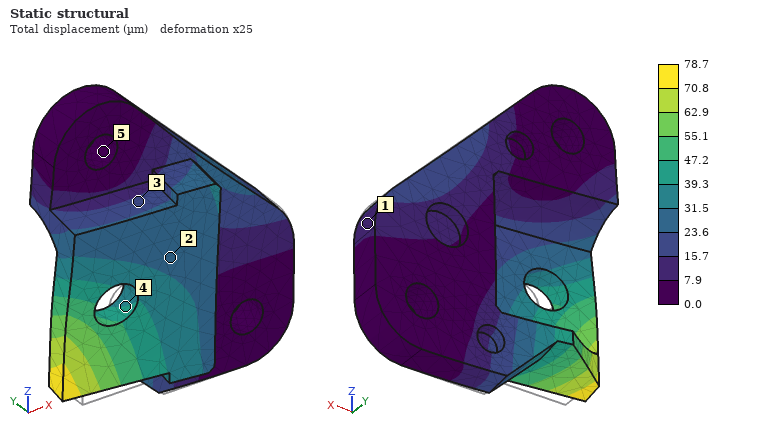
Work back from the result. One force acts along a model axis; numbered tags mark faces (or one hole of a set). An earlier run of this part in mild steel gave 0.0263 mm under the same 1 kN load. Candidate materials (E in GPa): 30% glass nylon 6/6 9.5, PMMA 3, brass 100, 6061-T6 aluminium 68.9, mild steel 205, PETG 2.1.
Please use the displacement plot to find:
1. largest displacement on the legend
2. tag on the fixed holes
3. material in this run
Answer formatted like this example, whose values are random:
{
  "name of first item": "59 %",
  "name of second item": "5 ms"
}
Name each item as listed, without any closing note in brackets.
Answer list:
{
  "largest displacement on the legend": "78.7 µm",
  "tag on the fixed holes": "5",
  "material in this run": "6061-T6 aluminium"
}
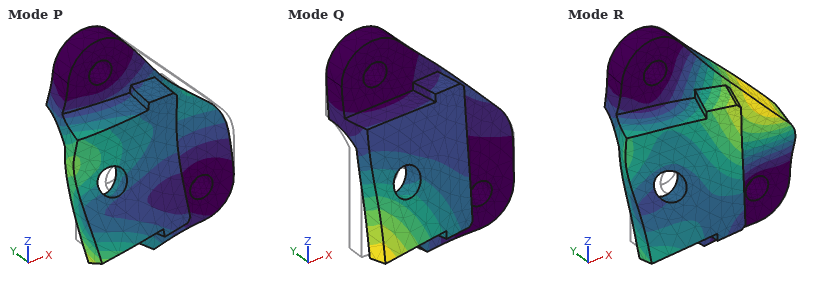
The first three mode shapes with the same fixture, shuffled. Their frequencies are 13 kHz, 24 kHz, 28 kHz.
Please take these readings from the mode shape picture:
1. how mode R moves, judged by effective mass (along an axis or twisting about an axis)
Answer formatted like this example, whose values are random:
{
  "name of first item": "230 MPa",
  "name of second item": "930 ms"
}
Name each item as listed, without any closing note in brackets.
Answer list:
{
  "how mode R moves, judged by effective mass": "along Y"
}
